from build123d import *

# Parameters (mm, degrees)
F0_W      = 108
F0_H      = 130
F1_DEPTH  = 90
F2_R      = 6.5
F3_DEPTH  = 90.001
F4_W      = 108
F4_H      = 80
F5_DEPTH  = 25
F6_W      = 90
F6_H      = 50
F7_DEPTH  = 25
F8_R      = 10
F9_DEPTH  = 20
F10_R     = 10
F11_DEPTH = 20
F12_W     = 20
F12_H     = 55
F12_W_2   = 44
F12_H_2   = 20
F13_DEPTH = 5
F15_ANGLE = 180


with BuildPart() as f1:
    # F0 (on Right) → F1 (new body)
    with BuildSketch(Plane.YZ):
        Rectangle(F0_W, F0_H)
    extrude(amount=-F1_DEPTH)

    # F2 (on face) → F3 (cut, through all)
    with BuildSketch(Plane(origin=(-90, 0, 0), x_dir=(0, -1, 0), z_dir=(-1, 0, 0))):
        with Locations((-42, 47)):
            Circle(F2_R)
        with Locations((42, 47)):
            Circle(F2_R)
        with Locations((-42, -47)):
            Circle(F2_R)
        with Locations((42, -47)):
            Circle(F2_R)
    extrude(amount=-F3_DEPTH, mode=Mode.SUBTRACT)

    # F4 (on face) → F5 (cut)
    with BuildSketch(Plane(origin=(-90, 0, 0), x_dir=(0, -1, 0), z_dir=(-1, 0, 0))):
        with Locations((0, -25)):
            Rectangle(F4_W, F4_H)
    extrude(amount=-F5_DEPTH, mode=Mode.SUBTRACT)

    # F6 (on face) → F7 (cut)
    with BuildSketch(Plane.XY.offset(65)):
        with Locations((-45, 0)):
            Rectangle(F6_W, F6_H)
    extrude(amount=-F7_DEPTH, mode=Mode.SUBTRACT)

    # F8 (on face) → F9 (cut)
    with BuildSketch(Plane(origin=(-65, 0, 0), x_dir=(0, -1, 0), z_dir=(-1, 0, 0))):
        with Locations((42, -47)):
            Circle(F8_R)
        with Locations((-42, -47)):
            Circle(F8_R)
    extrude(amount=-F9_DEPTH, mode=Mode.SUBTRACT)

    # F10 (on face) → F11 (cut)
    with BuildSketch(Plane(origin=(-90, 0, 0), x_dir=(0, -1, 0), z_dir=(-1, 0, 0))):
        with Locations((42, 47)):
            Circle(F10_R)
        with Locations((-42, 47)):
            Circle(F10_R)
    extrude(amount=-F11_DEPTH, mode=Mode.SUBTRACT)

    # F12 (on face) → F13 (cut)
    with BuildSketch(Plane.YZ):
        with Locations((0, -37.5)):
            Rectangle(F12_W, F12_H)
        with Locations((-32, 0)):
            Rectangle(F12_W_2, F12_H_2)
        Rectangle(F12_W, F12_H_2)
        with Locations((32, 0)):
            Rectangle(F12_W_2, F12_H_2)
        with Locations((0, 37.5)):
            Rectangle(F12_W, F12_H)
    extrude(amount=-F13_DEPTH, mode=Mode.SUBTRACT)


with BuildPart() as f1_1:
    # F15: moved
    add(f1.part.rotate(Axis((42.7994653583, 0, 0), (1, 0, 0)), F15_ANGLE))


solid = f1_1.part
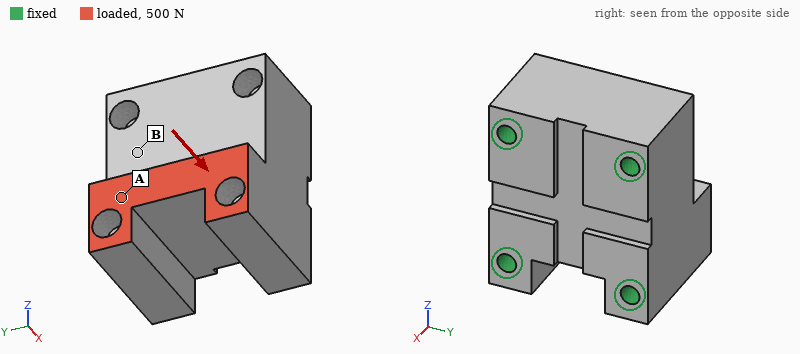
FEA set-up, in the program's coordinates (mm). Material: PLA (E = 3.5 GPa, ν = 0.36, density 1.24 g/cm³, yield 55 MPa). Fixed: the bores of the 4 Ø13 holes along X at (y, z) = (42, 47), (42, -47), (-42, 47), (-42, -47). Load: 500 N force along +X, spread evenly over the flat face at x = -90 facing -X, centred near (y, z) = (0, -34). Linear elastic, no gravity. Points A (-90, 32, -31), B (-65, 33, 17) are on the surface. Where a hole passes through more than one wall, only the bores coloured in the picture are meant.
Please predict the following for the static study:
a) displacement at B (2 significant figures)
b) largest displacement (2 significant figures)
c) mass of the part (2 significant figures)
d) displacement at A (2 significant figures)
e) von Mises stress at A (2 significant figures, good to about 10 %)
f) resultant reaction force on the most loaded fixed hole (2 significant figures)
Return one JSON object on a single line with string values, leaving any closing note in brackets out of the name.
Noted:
{"displacement at B": "0.56 µm", "largest displacement": "2.7 µm", "mass of the part": "1.1 kg", "displacement at A": "2.2 µm", "von Mises stress at A": "0.14 MPa", "resultant reaction force on the most loaded fixed hole": "220 N"}
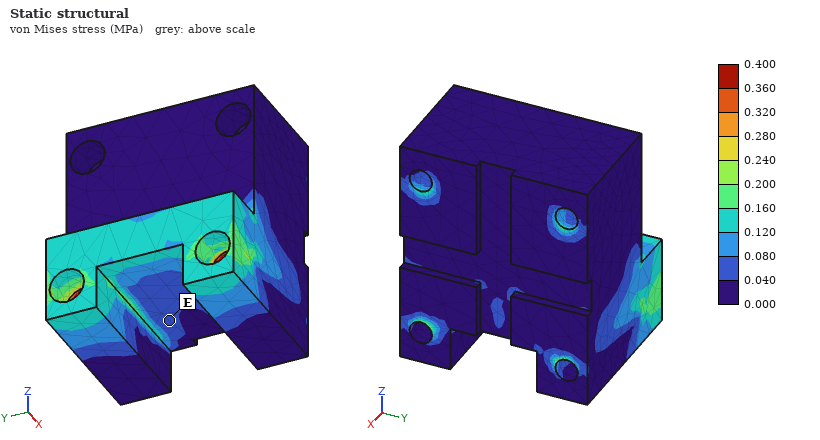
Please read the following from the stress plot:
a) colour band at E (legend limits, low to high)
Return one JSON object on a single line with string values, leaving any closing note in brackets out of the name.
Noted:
{"colour band at E": "0.040 to 0.080 MPa"}
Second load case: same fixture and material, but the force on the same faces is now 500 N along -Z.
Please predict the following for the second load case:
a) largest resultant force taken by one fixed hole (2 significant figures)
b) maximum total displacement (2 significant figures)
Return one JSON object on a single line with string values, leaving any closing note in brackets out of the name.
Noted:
{"largest resultant force taken by one fixed hole": "210 N", "maximum total displacement": "13 µm"}
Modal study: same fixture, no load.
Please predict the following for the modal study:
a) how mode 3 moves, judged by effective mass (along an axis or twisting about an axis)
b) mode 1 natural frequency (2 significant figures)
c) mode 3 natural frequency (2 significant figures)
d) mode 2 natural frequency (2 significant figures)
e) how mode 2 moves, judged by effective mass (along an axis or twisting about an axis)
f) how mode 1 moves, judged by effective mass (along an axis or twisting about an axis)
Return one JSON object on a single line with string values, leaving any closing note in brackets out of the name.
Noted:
{"how mode 3 moves, judged by effective mass": "along Z", "mode 1 natural frequency": "3600 Hz", "mode 3 natural frequency": "4600 Hz", "mode 2 natural frequency": "4000 Hz", "how mode 2 moves, judged by effective mass": "along Y", "how mode 1 moves, judged by effective mass": "along X"}
